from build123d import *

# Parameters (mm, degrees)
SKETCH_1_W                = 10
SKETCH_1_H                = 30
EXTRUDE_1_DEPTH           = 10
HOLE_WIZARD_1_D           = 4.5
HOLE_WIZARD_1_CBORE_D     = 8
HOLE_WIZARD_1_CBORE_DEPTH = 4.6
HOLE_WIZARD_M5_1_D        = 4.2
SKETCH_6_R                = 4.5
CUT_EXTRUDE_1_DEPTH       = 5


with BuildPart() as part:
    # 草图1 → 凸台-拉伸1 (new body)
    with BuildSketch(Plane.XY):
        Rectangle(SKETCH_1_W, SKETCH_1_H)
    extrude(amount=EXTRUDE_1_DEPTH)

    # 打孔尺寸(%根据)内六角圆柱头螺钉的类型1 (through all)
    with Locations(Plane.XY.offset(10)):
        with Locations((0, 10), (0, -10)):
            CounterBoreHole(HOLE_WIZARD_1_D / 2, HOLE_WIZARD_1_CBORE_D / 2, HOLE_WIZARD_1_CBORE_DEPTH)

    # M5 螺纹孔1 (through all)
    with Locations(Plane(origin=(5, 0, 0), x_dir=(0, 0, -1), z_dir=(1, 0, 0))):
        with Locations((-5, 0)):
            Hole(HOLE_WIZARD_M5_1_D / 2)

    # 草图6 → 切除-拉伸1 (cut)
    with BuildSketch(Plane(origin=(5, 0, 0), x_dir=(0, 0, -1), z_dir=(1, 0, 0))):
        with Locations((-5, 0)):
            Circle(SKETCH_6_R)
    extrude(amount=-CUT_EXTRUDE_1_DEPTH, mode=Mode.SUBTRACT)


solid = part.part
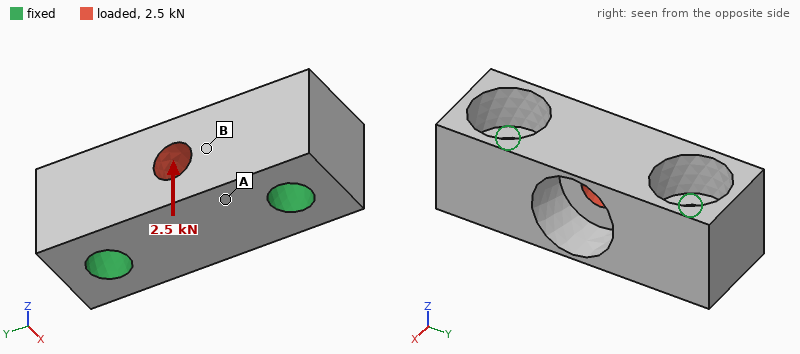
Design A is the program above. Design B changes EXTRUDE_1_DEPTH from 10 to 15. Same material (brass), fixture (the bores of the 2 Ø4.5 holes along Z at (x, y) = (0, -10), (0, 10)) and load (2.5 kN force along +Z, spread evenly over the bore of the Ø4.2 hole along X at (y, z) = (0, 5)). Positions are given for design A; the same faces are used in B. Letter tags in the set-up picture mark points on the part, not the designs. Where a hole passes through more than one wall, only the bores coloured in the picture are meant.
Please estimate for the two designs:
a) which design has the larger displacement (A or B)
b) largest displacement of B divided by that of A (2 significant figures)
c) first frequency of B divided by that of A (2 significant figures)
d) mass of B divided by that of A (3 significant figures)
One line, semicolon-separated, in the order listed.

A; 0.85; 0.52; 1.50
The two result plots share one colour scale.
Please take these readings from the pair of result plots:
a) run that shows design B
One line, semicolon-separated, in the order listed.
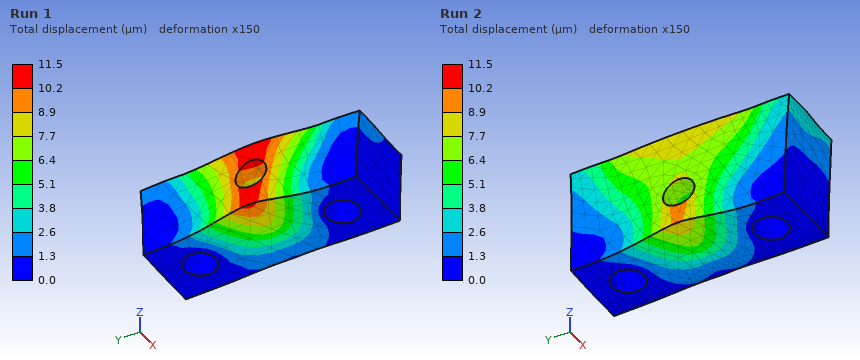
Run 2
